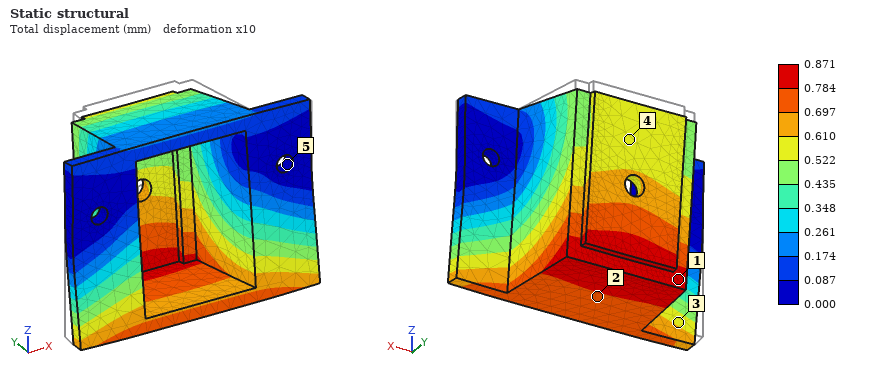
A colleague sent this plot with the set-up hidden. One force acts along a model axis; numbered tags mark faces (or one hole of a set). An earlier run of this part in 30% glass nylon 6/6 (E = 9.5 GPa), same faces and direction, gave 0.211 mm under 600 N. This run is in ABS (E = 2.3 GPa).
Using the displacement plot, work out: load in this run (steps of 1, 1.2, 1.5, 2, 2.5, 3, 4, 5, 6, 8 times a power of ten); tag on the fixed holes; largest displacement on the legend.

600 N
5
0.871 mm
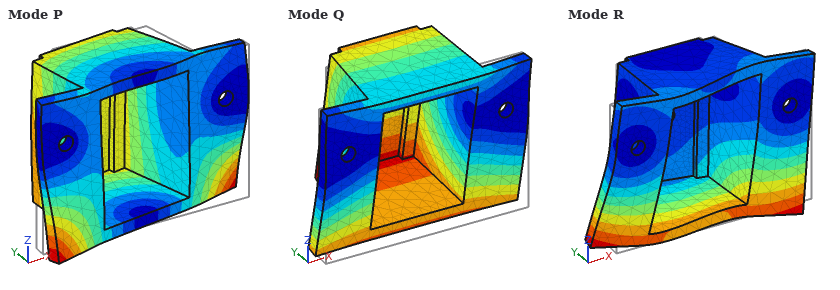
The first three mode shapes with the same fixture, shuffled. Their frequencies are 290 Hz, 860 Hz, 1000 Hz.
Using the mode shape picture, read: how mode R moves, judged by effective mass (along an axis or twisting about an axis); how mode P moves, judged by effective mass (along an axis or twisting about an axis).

along X
along X
